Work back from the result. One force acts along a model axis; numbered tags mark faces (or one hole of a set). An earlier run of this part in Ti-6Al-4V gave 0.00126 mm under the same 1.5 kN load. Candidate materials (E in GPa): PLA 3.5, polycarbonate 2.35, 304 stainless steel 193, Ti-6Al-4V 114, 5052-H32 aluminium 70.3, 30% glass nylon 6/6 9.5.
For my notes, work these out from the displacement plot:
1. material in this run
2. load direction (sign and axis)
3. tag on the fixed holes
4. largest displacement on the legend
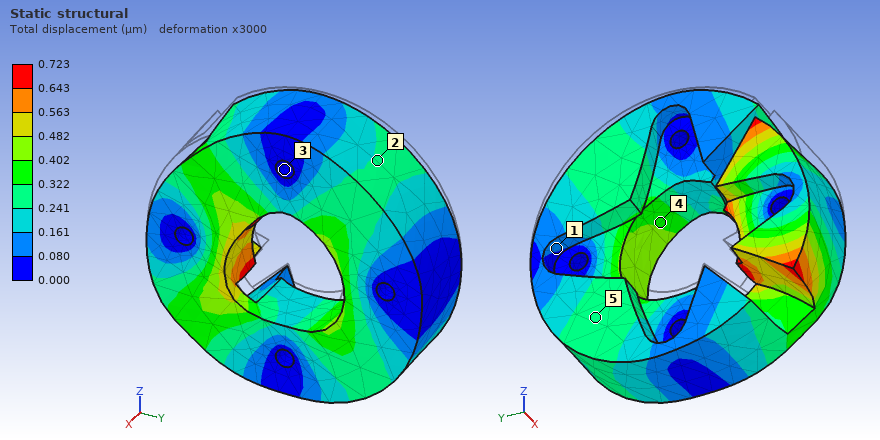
304 stainless steel
-Z
3
0.723 µm
